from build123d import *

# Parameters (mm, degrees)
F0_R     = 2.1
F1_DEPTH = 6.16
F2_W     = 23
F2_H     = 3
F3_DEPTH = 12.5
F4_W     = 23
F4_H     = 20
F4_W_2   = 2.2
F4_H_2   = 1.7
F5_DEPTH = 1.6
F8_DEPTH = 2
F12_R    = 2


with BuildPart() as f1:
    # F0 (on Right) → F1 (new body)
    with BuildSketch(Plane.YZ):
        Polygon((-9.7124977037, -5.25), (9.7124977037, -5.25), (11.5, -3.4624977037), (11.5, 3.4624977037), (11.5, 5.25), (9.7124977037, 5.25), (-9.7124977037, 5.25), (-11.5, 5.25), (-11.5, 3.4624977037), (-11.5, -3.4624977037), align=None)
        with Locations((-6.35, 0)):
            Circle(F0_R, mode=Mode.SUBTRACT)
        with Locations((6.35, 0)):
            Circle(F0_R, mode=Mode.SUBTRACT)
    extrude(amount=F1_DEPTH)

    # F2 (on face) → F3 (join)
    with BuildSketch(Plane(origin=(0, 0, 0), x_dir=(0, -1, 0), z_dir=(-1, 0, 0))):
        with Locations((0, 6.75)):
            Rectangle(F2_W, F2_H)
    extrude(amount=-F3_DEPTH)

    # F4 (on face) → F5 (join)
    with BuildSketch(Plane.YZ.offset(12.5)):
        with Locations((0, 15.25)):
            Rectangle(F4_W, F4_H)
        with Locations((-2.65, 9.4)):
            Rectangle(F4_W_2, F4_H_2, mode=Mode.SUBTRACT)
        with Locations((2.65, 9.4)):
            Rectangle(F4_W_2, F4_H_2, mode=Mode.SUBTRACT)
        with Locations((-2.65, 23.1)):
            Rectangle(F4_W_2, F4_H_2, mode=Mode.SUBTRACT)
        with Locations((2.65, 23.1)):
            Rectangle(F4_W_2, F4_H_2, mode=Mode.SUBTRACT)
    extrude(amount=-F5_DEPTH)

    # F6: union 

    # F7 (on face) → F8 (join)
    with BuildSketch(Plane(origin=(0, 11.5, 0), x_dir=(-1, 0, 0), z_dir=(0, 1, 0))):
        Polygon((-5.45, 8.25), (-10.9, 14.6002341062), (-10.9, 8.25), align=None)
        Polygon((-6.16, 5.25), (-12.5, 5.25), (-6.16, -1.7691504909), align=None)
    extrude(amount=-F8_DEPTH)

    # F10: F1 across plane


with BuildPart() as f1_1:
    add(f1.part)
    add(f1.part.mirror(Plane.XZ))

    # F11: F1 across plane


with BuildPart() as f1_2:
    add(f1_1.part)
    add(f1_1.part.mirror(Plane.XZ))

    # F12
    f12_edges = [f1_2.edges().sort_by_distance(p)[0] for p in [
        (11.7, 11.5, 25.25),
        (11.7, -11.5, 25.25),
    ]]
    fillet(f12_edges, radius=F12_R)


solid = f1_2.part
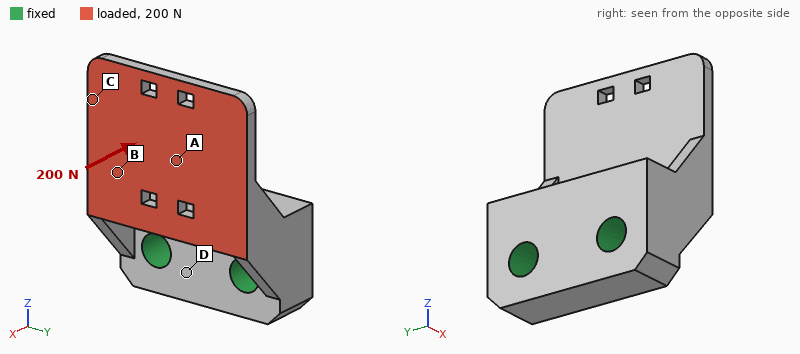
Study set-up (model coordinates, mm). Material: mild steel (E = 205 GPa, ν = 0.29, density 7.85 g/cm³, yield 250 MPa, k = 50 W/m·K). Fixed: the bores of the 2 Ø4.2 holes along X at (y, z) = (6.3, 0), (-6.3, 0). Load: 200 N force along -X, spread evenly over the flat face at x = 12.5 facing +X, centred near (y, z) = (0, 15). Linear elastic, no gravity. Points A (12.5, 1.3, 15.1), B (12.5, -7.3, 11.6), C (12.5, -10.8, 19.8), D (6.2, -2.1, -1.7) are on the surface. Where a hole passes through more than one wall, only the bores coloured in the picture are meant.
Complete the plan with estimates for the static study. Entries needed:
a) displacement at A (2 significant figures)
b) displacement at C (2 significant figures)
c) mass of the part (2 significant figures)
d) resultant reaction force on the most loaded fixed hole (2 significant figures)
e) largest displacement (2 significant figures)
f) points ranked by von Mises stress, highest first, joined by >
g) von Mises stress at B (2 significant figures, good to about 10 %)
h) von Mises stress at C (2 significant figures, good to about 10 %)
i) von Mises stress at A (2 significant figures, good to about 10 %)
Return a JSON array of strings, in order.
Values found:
["16 µm", "22 µm", "23 g", "110 N", "49 µm", "B > A > C > D", "60 MPa", "19 MPa", "36 MPa"]
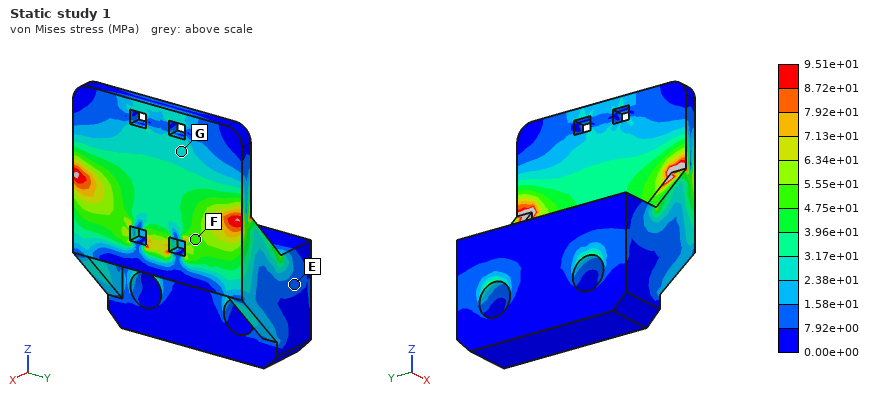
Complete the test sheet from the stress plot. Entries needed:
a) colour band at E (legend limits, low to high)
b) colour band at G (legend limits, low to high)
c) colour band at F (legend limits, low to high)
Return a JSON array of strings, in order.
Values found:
["7.92e+00 to 1.58e+01 MPa", "2.38e+01 to 3.17e+01 MPa", "4.75e+01 to 5.55e+01 MPa"]
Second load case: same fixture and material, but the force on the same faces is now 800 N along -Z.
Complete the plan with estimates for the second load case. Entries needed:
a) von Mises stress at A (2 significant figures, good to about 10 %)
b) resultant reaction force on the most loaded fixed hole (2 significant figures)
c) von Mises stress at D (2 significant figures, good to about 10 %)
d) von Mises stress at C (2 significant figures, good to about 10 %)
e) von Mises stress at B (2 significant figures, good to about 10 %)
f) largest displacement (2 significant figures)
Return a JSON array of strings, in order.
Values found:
["29 MPa", "400 N", "8.6 MPa", "26 MPa", "51 MPa", "46 µm"]
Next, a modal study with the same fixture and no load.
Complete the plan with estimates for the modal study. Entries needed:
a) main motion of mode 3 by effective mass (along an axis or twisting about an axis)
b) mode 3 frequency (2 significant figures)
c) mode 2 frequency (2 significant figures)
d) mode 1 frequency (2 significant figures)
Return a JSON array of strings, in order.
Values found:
["along Y", "20 kHz", "11 kHz", "5600 Hz"]
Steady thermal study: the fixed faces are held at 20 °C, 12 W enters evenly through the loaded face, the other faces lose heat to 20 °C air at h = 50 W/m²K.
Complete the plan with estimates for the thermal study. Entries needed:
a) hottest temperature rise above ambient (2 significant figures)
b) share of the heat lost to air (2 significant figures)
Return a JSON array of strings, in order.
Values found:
["63 K", "15 %"]
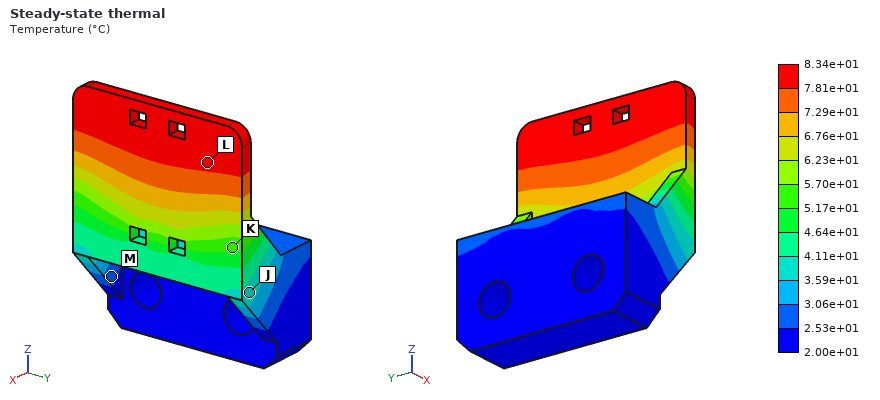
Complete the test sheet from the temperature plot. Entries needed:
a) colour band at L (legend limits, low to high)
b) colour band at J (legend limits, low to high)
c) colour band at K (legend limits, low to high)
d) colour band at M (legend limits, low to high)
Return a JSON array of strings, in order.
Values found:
["7.81e+01 to 8.34e+01 °C", "3.59e+01 to 4.11e+01 °C", "5.17e+01 to 5.70e+01 °C", "2.53e+01 to 3.06e+01 °C"]
